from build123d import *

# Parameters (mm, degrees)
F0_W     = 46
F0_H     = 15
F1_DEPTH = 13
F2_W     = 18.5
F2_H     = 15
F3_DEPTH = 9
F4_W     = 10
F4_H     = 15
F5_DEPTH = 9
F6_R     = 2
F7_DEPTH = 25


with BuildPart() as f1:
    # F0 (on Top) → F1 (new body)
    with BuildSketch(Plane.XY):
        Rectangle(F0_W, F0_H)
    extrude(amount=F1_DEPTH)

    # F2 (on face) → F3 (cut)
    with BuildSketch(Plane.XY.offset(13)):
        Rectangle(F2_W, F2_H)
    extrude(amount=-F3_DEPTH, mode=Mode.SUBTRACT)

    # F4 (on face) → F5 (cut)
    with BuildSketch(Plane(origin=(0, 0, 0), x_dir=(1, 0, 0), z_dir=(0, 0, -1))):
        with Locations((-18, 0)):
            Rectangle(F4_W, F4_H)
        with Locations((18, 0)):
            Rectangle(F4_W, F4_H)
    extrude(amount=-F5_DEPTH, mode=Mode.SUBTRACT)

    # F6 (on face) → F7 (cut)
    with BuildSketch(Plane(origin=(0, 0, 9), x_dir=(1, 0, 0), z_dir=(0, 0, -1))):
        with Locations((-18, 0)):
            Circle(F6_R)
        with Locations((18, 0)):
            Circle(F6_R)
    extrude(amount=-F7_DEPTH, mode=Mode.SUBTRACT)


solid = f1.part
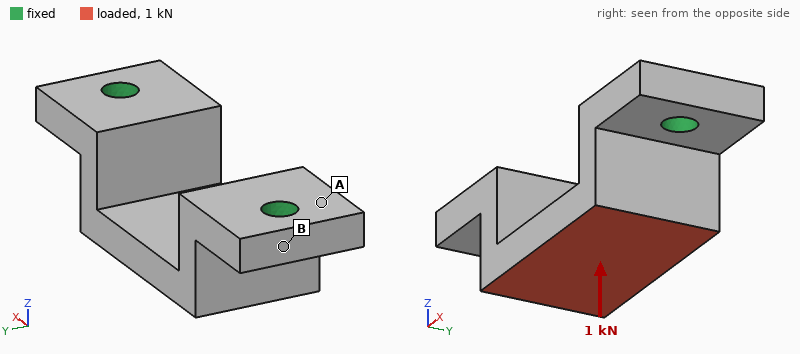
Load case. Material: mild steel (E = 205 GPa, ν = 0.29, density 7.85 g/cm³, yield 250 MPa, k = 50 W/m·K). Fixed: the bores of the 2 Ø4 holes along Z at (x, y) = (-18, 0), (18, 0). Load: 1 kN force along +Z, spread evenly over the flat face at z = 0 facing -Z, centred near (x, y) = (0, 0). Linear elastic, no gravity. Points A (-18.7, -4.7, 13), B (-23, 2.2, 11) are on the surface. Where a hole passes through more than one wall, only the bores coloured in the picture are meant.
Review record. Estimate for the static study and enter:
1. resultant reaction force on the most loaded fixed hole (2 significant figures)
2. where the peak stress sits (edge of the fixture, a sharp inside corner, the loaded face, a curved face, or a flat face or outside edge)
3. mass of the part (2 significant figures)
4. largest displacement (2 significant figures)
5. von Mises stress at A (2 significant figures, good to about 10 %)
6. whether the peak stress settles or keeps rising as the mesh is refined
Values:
590 N
edge of the fixture
29 g
4.3 µm
13 MPa
keeps rising
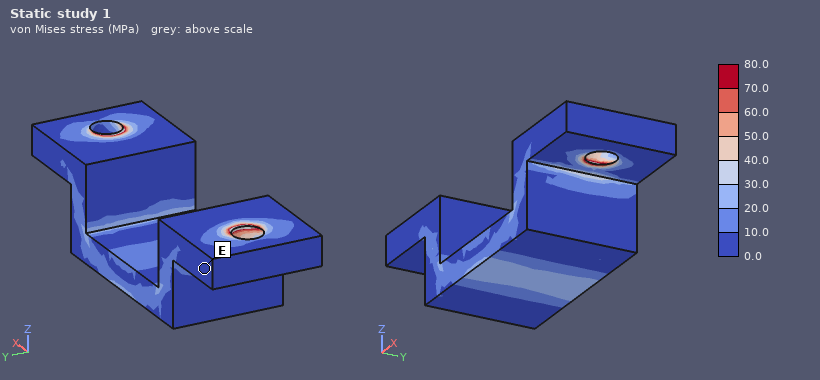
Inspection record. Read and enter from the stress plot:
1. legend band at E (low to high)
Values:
0.0 to 10.0 MPa
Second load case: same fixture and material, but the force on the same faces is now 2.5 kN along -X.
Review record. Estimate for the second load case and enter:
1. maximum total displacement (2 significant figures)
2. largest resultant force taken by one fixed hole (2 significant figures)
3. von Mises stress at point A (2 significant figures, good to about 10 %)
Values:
15 µm
1.5 kN
10 MPa
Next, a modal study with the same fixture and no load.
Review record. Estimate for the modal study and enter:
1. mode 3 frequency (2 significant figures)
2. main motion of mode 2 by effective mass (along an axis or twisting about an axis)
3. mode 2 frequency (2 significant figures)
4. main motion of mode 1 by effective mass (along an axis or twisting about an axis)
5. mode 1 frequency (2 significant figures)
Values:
21 kHz
along X
17 kHz
along Y
11 kHz
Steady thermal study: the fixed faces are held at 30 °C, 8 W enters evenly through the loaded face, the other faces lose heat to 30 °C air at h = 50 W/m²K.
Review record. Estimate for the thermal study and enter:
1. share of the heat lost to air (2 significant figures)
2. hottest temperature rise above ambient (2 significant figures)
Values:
12 %
22 K
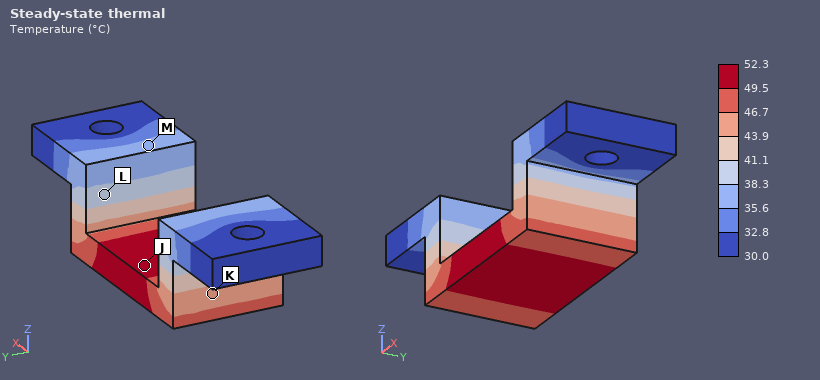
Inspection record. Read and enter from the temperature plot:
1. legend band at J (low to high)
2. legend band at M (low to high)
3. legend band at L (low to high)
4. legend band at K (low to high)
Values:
49.5 to 52.3 °C
35.6 to 38.3 °C
38.3 to 41.1 °C
43.9 to 46.7 °C
